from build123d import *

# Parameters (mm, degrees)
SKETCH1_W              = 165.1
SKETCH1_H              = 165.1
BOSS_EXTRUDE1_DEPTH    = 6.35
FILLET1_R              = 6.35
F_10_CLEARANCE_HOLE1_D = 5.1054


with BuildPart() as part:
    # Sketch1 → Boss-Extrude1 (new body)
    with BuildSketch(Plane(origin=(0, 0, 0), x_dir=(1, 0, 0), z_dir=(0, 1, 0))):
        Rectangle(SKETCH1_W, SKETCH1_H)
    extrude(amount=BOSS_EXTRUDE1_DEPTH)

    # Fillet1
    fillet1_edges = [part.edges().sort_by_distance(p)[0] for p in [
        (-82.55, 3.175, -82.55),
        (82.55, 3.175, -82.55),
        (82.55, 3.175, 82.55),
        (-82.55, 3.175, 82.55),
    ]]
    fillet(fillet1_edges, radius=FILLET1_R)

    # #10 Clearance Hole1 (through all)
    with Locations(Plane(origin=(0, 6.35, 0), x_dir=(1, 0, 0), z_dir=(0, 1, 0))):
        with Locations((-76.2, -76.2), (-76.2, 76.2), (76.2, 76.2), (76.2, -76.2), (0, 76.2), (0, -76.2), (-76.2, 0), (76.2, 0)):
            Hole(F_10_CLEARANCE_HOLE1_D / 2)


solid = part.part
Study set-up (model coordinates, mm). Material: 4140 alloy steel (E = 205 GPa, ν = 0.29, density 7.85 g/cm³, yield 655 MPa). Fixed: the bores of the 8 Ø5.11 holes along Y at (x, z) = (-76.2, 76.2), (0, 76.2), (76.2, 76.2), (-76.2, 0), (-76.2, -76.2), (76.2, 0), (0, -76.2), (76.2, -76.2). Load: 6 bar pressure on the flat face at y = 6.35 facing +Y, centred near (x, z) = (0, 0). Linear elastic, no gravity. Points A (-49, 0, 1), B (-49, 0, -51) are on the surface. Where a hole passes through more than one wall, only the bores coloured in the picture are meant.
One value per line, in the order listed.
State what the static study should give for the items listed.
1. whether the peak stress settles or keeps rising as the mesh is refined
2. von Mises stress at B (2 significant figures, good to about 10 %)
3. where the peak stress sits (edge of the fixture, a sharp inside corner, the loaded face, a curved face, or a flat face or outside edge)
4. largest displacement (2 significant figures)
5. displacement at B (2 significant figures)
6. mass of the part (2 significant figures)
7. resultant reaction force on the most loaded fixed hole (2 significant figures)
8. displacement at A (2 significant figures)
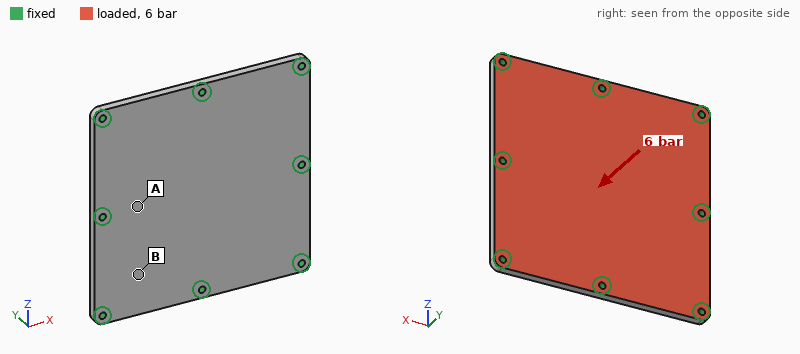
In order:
keeps rising
34 MPa
edge of the fixture
0.13 mm
0.046 mm
1.3 kg
3.1 kN
0.063 mm
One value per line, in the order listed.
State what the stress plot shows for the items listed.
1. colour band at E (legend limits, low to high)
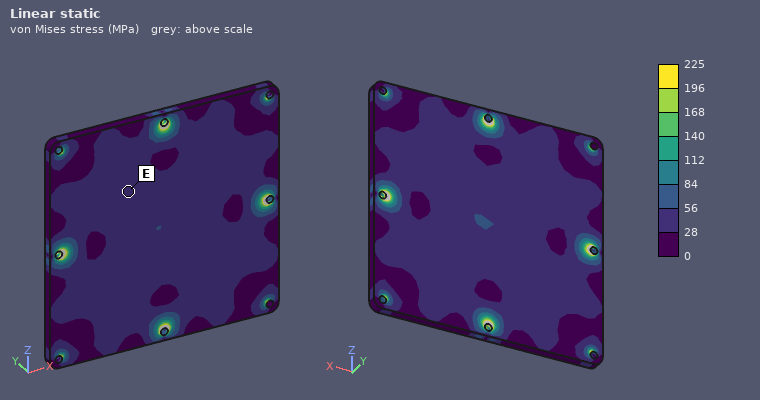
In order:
28 to 56 MPa
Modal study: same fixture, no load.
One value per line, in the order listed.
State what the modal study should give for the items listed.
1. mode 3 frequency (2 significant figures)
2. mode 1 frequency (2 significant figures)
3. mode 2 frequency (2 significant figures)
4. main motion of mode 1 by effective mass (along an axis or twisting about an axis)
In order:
3400 Hz
1900 Hz
3400 Hz
along Y
